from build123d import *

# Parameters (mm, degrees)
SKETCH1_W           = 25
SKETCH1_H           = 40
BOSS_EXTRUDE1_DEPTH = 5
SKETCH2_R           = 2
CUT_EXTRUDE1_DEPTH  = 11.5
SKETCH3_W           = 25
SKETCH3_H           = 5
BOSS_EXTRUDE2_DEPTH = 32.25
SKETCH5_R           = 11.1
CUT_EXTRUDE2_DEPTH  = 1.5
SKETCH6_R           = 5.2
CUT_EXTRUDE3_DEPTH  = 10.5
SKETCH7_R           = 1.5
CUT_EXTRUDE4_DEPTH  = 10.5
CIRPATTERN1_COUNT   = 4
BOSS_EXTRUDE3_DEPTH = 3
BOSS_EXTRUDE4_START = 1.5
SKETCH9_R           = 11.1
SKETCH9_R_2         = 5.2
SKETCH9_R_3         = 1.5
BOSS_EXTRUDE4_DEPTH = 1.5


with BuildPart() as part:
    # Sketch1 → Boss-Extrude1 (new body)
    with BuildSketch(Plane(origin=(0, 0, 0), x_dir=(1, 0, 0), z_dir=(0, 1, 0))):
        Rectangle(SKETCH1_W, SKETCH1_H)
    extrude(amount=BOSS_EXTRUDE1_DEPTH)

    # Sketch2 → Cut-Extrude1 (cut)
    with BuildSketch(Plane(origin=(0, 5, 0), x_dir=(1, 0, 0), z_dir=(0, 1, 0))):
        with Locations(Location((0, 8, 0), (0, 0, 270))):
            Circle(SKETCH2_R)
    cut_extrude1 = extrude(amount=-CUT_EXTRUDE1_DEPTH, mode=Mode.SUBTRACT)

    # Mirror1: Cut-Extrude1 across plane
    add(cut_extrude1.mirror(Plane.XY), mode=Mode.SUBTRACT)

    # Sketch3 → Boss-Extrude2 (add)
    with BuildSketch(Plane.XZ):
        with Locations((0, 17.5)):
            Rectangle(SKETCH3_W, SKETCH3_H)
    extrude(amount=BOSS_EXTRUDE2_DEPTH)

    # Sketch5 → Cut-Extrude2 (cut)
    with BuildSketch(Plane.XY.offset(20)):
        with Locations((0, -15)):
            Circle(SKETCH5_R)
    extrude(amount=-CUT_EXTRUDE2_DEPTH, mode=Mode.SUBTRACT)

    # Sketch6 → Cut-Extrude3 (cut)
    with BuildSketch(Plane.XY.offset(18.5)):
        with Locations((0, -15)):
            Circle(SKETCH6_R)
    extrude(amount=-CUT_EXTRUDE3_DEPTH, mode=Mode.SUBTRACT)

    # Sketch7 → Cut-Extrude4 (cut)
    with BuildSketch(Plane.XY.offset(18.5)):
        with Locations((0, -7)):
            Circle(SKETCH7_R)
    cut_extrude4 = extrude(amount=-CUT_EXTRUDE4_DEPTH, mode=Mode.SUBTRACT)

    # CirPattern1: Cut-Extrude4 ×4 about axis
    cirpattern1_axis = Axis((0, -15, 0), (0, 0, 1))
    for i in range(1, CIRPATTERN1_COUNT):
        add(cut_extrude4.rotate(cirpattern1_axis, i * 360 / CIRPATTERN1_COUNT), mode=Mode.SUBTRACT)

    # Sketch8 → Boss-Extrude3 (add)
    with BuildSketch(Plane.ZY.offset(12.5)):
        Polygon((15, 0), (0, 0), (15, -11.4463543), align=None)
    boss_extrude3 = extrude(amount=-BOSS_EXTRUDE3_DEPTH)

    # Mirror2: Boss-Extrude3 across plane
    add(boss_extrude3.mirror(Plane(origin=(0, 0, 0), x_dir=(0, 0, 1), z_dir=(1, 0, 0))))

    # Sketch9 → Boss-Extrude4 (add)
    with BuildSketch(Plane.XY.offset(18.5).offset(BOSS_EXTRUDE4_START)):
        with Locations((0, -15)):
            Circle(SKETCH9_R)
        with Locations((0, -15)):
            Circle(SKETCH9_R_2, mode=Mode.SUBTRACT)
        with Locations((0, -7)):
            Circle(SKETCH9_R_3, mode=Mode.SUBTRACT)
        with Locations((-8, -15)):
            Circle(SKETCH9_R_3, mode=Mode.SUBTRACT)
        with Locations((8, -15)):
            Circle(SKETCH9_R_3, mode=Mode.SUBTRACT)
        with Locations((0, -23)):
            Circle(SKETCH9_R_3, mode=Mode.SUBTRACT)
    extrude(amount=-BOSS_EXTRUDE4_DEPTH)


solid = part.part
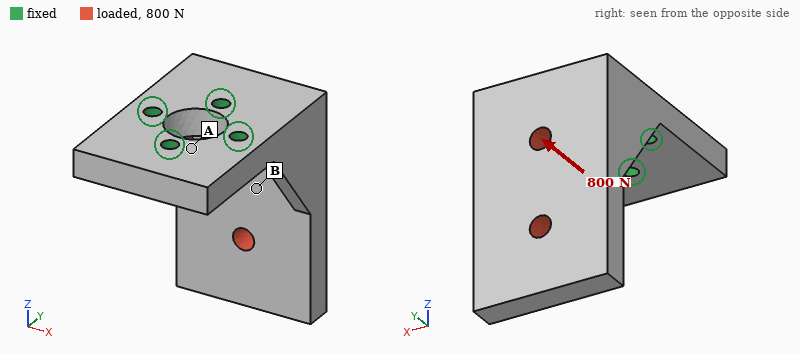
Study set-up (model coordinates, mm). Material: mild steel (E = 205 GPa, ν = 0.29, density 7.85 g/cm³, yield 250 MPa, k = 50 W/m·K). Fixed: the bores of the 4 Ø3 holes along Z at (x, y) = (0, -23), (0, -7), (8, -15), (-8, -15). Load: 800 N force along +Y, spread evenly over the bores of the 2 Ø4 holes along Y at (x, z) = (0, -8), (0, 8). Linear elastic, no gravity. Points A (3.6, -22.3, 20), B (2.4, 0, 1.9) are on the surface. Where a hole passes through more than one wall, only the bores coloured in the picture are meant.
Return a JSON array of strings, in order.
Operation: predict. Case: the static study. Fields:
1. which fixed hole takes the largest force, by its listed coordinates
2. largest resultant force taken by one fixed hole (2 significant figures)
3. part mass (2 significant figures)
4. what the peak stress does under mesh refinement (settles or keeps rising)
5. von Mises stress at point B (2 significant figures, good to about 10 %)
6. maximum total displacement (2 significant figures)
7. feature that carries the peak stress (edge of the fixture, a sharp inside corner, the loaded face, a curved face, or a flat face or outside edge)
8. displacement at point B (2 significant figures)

["(0, -7)", "1.1 kN", "70 g", "keeps rising", "34 MPa", "64 µm", "edge of the fixture", "22 µm"]
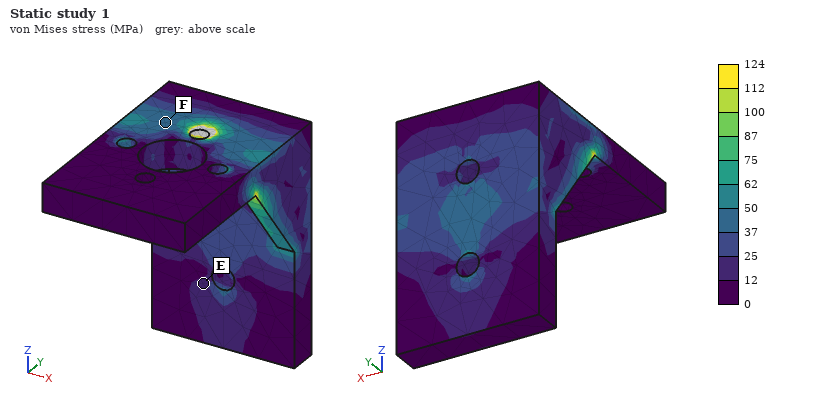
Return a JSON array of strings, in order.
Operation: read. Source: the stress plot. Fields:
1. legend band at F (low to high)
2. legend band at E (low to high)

["37 to 50 MPa", "12 to 25 MPa"]
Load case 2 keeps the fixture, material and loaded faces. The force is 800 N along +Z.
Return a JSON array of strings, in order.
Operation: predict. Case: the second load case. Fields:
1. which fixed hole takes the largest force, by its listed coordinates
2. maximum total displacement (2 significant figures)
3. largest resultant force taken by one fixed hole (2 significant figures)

["(0, -7)", "21 µm", "1.0 kN"]
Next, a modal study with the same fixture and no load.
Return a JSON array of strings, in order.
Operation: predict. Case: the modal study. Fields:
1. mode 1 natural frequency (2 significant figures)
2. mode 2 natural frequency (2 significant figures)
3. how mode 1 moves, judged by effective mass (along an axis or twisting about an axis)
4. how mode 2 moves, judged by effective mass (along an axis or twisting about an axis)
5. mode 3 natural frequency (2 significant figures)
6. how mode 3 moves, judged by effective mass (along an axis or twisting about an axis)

["3400 Hz", "4100 Hz", "along Y", "along X", "10 kHz", "along Z"]
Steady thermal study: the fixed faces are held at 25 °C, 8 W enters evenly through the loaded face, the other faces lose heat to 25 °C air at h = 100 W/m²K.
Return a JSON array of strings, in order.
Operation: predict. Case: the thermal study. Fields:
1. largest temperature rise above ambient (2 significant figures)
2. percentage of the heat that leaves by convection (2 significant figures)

["19 K", "45 %"]
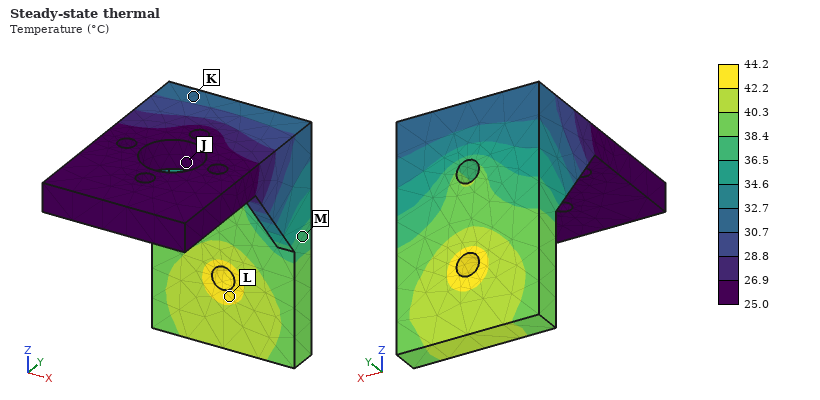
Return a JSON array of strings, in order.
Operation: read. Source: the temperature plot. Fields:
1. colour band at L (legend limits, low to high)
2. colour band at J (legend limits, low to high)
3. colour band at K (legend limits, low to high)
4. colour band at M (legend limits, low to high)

["42.2 to 44.2 °C", "25.0 to 26.9 °C", "30.7 to 32.7 °C", "36.5 to 38.4 °C"]
